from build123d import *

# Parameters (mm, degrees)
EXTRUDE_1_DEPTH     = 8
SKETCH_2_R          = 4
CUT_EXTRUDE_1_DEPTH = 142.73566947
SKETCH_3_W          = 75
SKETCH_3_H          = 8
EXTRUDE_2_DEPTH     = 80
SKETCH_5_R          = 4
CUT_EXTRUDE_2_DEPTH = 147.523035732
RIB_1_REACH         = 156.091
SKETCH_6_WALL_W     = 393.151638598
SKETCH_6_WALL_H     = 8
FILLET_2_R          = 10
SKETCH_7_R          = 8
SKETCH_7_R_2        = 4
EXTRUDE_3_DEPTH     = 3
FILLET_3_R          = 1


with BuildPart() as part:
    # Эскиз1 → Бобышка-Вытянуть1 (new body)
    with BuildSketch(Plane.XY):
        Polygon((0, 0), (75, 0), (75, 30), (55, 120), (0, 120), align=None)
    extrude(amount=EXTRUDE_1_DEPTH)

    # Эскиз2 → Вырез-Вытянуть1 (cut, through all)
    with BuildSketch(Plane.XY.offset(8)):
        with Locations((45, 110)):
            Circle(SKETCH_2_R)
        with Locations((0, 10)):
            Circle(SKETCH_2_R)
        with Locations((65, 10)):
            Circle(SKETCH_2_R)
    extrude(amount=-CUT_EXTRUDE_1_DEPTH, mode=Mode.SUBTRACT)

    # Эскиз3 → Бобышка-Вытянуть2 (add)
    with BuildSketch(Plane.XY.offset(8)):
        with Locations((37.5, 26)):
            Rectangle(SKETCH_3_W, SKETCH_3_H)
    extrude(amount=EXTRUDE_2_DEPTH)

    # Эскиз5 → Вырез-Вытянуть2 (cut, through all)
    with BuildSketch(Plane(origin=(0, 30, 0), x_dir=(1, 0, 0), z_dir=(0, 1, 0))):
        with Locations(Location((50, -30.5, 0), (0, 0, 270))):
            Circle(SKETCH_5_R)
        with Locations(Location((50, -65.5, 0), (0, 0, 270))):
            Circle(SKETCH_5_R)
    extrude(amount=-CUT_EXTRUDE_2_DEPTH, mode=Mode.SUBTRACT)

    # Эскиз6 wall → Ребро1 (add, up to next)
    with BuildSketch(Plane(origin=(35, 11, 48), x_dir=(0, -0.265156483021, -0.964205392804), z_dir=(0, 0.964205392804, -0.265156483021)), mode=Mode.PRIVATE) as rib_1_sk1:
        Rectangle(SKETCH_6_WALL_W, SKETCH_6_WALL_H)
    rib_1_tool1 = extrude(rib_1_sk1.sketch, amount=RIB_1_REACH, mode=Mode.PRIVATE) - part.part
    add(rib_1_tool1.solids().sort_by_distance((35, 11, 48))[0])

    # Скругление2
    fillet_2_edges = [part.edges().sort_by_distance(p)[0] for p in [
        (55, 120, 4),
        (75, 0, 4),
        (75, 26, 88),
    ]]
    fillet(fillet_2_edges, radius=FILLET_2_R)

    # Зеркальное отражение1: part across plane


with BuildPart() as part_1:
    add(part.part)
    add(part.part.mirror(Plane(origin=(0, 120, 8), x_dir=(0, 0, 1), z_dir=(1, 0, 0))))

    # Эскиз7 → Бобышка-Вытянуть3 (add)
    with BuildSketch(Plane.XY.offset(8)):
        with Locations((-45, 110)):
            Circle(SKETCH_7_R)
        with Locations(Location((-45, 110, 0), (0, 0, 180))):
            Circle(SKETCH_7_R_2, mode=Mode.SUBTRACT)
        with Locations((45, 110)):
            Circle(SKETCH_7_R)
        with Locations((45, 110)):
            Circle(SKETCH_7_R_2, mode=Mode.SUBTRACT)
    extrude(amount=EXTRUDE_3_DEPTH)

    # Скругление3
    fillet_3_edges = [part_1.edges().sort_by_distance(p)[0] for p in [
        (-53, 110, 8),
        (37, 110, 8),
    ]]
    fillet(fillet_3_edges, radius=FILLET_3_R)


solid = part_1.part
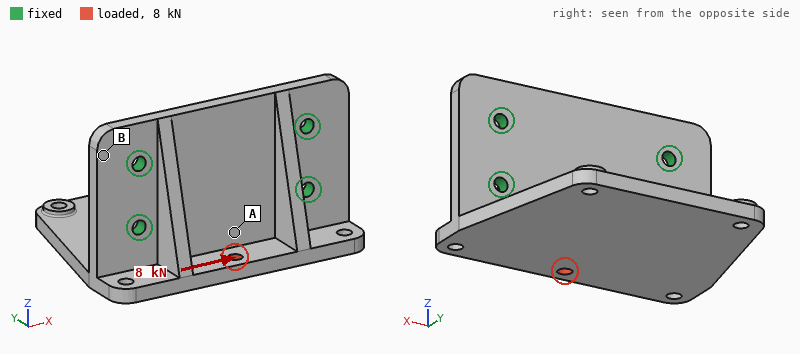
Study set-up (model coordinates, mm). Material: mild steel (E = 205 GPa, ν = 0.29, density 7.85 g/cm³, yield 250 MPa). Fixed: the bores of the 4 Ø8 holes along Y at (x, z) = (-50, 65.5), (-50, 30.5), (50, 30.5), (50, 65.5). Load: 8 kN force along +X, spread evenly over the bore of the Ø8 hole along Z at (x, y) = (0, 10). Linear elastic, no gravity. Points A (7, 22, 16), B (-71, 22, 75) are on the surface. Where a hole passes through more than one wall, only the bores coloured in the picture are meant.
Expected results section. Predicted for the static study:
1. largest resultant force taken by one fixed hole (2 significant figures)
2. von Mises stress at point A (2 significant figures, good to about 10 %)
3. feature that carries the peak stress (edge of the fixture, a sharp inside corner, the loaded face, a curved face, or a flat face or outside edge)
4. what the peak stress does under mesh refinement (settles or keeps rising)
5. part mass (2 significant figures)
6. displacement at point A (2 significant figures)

4.3 kN
19 MPa
edge of the fixture
keeps rising
1.9 kg
2.8 µm
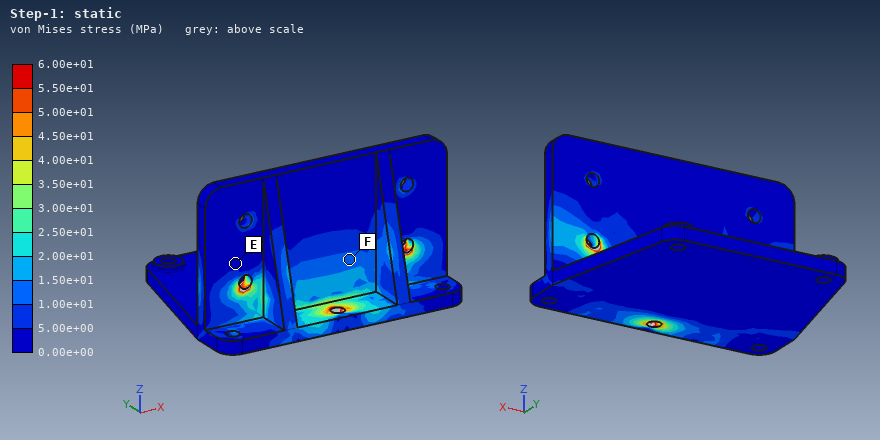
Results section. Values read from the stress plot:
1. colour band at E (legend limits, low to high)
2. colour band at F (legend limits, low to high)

0.00e+00 to 5.00e+00 MPa
1.00e+01 to 1.50e+01 MPa
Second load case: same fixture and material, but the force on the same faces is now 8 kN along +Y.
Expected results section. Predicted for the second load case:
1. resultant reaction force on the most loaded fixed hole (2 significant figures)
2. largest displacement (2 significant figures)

5.9 kN
0.10 mm
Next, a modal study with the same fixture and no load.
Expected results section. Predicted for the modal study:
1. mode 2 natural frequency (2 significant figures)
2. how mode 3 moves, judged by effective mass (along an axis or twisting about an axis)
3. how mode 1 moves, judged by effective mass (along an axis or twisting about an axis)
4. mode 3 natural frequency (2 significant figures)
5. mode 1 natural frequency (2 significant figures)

1500 Hz
along X
along Z
2400 Hz
700 Hz
